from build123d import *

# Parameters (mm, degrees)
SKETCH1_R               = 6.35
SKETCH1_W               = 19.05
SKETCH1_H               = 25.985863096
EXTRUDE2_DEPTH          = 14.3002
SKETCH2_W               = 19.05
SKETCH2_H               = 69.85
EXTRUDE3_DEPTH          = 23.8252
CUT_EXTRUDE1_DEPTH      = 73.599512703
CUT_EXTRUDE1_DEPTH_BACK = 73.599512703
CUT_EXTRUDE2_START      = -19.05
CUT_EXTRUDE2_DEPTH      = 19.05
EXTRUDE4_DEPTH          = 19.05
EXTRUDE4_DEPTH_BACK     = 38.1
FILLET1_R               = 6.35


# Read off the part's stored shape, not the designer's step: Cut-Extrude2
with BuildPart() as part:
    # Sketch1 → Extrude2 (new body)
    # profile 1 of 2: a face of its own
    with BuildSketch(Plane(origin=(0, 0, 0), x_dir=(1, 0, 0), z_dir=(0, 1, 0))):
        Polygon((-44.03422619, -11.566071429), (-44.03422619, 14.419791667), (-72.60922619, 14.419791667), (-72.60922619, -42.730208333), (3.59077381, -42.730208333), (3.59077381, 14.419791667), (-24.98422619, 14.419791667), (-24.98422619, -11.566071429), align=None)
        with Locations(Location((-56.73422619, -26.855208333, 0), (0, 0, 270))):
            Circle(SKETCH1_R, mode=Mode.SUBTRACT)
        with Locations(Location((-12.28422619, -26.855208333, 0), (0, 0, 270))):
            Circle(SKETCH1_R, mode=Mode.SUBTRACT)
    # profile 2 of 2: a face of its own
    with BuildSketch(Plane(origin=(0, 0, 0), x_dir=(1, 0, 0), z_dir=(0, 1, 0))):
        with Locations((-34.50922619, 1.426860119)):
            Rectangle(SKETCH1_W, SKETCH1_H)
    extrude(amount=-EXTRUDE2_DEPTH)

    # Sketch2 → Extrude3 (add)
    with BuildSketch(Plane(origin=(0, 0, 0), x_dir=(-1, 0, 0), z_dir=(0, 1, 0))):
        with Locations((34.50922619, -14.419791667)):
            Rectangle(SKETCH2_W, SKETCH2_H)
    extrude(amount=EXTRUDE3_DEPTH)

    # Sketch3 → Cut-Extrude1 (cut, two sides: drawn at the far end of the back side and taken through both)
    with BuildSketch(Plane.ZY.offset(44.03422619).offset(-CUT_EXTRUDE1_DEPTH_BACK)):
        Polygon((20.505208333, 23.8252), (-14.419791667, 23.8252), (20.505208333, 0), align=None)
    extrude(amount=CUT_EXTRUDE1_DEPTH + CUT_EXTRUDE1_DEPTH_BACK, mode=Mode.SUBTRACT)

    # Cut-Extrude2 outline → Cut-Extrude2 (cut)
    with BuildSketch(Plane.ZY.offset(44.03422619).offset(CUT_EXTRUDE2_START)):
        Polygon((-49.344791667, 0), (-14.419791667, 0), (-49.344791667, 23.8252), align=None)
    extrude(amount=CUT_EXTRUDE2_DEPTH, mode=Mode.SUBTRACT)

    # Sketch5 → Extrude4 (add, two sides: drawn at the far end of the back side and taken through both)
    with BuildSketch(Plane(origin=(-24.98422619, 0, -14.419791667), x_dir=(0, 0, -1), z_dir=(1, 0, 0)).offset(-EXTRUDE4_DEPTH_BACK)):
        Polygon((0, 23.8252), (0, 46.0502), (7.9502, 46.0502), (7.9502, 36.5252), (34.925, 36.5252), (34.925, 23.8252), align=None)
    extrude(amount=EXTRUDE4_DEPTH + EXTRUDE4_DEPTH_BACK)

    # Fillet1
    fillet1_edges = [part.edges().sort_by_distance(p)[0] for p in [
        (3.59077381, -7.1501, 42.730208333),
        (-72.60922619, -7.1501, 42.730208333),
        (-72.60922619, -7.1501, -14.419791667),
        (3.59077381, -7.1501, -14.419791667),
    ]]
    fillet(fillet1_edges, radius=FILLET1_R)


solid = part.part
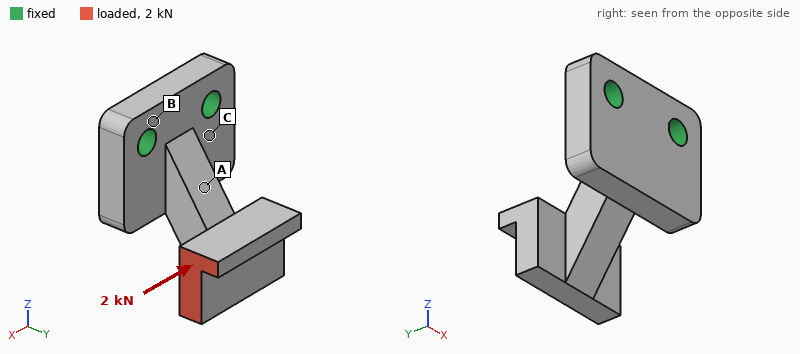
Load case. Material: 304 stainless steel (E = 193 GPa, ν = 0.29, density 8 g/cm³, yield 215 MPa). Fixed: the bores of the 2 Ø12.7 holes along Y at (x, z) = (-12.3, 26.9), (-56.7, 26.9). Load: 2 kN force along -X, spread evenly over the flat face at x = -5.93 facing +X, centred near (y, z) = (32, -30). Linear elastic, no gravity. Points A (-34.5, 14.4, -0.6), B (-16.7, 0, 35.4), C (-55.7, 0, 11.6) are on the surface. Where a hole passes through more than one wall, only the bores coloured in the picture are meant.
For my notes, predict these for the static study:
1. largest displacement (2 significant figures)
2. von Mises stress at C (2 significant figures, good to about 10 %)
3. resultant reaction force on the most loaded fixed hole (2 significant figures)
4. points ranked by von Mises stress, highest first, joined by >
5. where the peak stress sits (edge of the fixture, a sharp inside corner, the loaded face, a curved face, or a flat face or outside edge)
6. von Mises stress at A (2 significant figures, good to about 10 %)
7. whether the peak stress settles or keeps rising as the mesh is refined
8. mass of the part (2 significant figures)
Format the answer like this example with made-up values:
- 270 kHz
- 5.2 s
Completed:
- 60 µm
- 10 MPa
- 3.0 kN
- A > C > B
- a sharp inside corner
- 18 MPa
- keeps rising
- 830 g
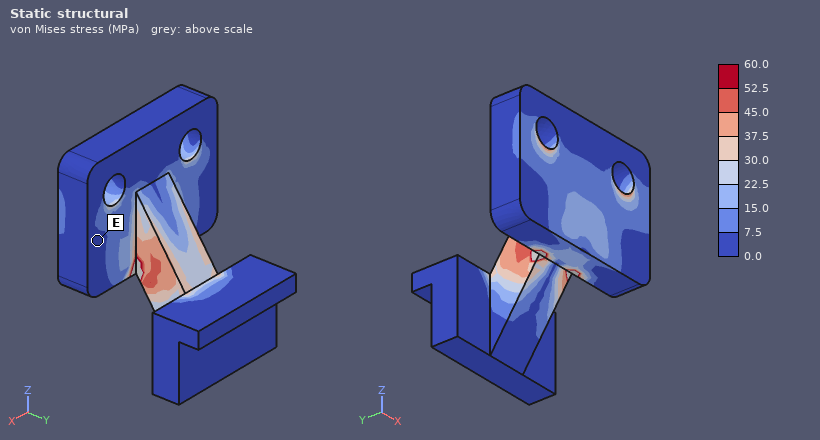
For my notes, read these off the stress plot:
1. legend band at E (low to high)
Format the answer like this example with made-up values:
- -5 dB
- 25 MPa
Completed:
- 0.0 to 7.5 MPa
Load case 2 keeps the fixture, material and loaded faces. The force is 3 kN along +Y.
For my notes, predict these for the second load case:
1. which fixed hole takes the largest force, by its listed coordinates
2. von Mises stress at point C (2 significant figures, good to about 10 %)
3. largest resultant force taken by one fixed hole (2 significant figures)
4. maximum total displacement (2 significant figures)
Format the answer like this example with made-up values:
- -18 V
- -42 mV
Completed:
- (-12.3, 26.9)
- 37 MPa
- 3.5 kN
- 0.16 mm
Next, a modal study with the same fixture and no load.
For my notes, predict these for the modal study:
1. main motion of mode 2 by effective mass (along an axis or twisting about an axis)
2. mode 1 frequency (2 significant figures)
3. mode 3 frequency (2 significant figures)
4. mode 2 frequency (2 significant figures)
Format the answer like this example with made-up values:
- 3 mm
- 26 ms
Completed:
- along X
- 1600 Hz
- 3500 Hz
- 2000 Hz
